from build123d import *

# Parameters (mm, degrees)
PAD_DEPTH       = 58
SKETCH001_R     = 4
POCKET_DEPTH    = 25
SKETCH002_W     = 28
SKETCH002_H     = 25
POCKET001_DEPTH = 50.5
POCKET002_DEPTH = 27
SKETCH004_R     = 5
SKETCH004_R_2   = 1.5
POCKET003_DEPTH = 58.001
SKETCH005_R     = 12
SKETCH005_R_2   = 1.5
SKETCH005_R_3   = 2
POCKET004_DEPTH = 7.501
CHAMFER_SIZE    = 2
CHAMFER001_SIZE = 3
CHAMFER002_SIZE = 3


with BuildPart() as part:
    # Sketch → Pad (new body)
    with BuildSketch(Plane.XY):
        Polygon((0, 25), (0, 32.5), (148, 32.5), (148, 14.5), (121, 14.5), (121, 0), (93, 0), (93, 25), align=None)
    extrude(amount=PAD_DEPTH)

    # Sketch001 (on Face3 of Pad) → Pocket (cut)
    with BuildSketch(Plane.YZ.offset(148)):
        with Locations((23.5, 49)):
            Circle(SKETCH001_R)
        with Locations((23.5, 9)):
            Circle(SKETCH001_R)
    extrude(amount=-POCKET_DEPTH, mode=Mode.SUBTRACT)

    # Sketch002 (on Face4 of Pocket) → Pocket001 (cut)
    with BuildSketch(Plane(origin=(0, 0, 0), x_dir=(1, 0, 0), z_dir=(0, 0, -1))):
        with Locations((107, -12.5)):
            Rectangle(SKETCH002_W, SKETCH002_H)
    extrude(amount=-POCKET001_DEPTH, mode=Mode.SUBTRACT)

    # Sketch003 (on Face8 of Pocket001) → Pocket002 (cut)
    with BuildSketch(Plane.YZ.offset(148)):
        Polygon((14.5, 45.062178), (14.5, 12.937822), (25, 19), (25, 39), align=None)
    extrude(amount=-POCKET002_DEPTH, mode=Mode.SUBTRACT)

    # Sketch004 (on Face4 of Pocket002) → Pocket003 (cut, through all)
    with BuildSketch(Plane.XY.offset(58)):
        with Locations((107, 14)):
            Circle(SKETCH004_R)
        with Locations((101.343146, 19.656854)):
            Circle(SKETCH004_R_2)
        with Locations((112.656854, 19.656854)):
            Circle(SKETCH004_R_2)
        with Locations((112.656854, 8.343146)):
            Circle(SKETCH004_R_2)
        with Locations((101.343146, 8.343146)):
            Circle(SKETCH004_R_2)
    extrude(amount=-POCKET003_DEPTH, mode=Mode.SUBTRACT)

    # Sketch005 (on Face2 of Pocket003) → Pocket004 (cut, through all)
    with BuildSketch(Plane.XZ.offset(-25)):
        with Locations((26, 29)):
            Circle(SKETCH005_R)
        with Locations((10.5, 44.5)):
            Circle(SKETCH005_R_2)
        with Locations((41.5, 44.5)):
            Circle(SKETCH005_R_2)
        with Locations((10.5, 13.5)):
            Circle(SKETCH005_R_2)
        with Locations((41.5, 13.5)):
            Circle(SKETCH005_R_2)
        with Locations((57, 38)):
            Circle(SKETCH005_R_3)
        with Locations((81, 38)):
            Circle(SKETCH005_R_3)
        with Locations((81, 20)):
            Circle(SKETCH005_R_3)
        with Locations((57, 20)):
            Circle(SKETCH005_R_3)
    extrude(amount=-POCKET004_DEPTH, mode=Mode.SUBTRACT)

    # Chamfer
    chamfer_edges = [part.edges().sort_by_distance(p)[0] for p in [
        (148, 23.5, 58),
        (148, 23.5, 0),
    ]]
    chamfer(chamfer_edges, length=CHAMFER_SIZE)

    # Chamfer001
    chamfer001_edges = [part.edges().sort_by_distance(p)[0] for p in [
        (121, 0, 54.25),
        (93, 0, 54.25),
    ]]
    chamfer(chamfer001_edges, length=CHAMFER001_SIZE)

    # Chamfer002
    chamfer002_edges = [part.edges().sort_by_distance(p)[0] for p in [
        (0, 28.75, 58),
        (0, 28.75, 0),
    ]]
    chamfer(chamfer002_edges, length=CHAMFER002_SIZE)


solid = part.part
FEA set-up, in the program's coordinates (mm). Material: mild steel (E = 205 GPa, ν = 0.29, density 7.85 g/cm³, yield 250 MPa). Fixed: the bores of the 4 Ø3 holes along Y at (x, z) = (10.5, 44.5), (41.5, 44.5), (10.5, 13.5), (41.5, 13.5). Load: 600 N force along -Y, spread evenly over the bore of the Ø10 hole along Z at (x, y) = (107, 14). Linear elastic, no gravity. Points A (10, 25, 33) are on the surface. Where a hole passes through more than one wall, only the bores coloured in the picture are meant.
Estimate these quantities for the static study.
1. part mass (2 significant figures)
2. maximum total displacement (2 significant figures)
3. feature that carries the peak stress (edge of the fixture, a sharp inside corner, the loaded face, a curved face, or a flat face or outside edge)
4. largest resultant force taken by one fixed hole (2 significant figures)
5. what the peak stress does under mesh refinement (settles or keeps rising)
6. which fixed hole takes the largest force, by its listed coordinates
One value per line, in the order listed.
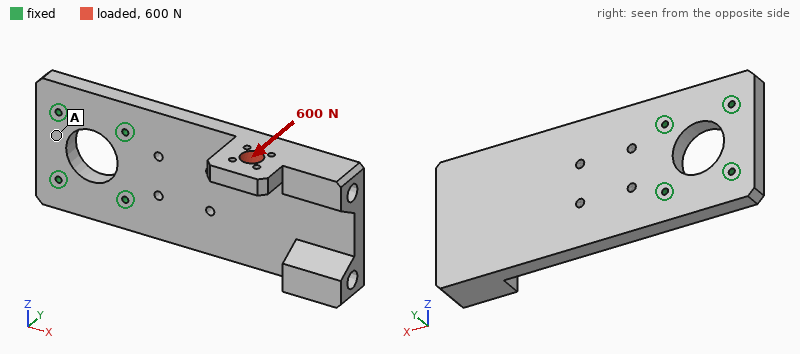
560 g
0.35 mm
edge of the fixture
960 N
keeps rising
(41.5, 44.5)
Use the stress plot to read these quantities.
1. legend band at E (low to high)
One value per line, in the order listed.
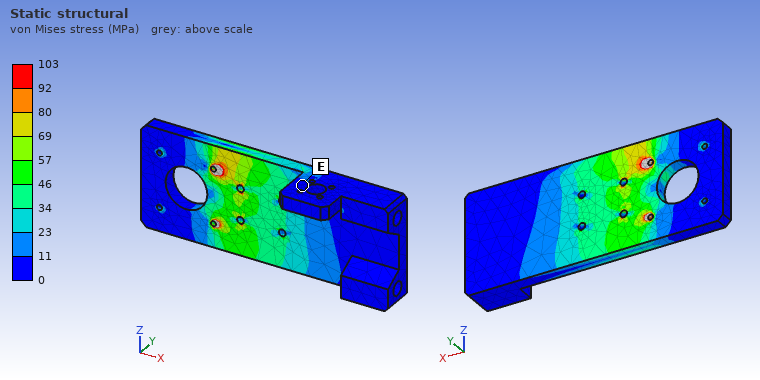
0 to 11 MPa
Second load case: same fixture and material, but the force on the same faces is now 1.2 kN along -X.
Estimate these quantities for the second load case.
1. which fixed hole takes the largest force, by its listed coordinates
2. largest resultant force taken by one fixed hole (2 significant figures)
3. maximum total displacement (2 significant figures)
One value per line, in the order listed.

(41.5, 44.5)
1.2 kN
0.24 mm
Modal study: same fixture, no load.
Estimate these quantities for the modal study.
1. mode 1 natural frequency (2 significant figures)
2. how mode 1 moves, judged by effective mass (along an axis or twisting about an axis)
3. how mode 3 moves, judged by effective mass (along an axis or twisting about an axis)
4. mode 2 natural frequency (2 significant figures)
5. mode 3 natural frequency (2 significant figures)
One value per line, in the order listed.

420 Hz
along Y
along Z
1500 Hz
2600 Hz
